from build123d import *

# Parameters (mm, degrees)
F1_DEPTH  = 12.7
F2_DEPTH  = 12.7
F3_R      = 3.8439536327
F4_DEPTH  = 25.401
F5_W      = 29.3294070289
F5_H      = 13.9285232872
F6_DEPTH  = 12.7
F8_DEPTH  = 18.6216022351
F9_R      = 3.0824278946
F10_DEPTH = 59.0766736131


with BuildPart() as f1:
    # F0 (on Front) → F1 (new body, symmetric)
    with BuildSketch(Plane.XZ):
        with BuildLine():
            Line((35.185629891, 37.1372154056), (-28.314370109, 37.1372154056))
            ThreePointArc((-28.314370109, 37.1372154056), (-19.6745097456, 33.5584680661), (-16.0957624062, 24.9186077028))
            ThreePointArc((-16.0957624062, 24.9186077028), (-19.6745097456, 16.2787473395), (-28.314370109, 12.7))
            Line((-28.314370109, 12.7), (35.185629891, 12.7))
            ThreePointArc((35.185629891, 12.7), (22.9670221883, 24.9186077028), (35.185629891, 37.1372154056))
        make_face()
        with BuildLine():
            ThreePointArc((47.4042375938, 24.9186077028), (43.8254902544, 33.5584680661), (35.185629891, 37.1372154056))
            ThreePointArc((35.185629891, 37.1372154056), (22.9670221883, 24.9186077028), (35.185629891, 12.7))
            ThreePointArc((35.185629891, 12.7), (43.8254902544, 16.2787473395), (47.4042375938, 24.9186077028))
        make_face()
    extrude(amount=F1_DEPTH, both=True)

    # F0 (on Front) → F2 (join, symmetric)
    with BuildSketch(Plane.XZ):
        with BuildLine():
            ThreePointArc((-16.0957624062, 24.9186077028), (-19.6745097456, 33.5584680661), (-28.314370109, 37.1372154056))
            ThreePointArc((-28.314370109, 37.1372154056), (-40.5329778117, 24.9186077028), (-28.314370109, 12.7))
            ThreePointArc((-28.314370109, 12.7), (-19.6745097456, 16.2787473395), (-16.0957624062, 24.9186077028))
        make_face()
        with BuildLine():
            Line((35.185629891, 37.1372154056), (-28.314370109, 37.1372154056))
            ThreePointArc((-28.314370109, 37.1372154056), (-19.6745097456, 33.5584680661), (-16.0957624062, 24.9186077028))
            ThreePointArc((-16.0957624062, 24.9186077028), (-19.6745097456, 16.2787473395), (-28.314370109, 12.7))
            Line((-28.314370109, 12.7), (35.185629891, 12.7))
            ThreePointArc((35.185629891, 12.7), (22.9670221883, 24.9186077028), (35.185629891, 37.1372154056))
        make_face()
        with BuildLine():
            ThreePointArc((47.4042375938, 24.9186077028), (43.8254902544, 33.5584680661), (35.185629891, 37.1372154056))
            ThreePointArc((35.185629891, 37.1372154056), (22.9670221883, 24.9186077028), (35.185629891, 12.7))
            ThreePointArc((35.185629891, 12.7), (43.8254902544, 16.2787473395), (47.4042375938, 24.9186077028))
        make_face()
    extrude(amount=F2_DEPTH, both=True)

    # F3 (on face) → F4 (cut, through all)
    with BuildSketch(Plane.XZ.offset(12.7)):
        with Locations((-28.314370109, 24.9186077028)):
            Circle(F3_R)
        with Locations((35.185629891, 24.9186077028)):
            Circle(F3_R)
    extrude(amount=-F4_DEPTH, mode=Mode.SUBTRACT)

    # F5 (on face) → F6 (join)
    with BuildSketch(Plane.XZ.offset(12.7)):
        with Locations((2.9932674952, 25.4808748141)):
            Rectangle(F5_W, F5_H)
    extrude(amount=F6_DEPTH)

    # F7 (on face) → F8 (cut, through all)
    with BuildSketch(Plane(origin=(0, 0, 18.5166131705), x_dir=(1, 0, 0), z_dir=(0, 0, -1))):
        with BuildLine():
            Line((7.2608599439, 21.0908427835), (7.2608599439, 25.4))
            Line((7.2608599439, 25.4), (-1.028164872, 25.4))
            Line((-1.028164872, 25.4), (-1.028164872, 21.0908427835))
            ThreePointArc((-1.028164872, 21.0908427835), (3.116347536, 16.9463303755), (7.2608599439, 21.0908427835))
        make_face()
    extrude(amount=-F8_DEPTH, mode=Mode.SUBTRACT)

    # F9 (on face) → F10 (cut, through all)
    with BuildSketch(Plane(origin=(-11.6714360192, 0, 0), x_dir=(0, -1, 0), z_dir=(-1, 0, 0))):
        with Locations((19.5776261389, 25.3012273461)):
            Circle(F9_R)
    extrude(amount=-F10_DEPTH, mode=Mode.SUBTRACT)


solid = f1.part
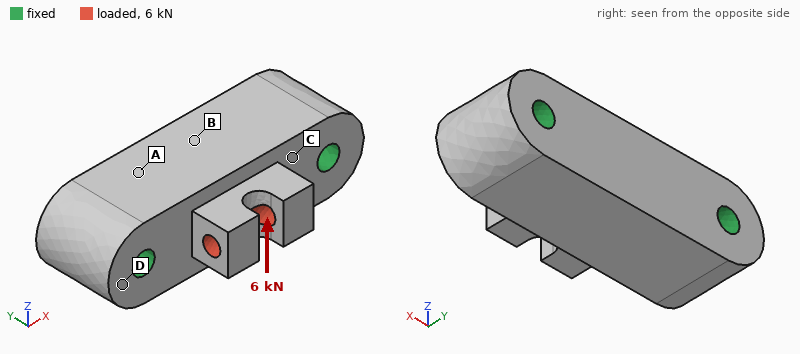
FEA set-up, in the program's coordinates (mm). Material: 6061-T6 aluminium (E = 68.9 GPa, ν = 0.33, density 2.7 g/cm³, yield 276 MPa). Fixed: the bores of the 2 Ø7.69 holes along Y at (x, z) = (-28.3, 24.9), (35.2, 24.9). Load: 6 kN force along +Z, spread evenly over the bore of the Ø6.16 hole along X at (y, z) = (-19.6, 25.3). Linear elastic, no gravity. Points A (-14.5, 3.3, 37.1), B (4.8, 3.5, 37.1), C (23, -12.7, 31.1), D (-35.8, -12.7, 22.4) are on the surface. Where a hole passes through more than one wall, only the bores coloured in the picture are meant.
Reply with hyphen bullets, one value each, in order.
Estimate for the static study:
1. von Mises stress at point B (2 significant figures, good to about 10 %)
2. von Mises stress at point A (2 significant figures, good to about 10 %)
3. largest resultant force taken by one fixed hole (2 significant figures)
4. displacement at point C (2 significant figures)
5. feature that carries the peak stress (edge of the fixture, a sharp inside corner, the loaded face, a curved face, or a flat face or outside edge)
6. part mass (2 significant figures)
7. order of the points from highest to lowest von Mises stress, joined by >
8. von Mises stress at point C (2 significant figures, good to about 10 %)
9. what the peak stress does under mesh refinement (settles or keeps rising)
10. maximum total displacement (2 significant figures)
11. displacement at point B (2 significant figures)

- 18 MPa
- 26 MPa
- 3.1 kN
- 12 µm
- edge of the fixture
- 140 g
- C > A > B > D
- 40 MPa
- keeps rising
- 57 µm
- 12 µm
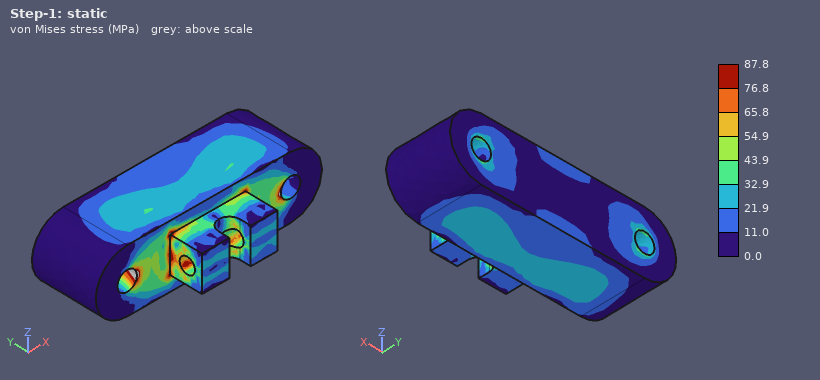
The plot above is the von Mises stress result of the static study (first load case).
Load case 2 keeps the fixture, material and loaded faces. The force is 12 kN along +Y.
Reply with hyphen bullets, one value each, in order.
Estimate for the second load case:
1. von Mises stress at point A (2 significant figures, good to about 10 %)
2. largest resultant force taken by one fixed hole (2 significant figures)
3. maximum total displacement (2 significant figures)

- 21 MPa
- 6.2 kN
- 25 µm
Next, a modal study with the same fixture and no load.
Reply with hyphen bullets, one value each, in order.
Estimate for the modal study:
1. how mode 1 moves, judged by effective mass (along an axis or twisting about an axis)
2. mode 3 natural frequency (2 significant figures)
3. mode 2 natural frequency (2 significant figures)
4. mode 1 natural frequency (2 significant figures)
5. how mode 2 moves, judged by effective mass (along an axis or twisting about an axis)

- along Z
- 19 kHz
- 18 kHz
- 14 kHz
- along Y
